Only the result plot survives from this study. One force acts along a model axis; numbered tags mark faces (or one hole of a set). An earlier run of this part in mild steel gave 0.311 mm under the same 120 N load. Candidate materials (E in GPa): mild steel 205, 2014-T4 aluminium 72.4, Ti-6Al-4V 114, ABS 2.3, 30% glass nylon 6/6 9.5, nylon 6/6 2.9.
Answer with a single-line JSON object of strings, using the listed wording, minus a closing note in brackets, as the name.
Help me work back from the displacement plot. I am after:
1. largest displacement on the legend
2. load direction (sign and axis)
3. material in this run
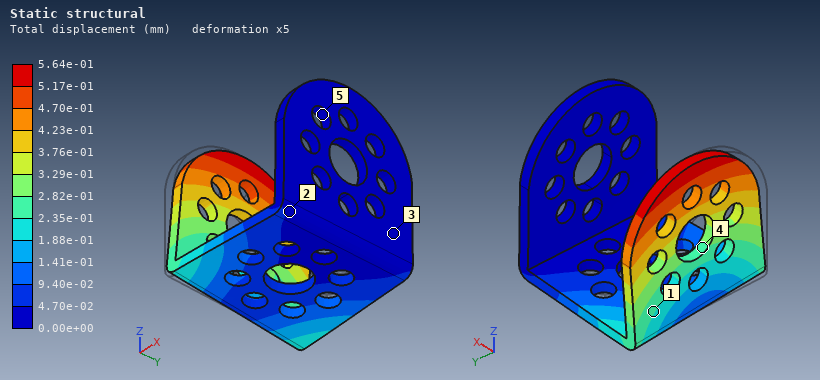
{"largest displacement on the legend": "5.64e-01 mm", "load direction": "+Y", "material in this run": "Ti-6Al-4V"}
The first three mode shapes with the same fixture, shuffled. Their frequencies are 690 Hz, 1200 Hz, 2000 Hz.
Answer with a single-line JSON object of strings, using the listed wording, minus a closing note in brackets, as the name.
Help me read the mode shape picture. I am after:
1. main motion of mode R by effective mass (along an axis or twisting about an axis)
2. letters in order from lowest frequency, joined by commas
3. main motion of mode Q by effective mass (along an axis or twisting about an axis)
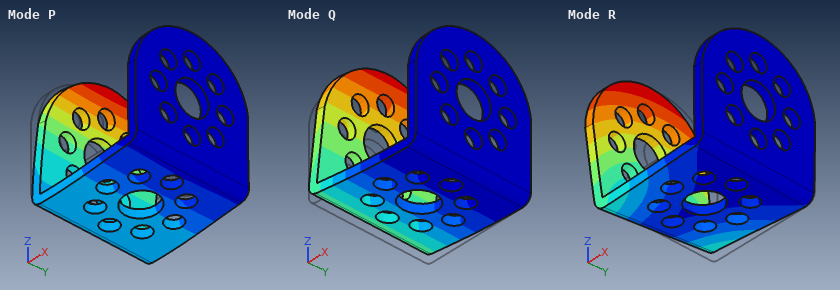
{"main motion of mode R by effective mass": "along Y", "letters in order from lowest frequency, joined by commas": "Q, R, P", "main motion of mode Q by effective mass": "along Z"}
